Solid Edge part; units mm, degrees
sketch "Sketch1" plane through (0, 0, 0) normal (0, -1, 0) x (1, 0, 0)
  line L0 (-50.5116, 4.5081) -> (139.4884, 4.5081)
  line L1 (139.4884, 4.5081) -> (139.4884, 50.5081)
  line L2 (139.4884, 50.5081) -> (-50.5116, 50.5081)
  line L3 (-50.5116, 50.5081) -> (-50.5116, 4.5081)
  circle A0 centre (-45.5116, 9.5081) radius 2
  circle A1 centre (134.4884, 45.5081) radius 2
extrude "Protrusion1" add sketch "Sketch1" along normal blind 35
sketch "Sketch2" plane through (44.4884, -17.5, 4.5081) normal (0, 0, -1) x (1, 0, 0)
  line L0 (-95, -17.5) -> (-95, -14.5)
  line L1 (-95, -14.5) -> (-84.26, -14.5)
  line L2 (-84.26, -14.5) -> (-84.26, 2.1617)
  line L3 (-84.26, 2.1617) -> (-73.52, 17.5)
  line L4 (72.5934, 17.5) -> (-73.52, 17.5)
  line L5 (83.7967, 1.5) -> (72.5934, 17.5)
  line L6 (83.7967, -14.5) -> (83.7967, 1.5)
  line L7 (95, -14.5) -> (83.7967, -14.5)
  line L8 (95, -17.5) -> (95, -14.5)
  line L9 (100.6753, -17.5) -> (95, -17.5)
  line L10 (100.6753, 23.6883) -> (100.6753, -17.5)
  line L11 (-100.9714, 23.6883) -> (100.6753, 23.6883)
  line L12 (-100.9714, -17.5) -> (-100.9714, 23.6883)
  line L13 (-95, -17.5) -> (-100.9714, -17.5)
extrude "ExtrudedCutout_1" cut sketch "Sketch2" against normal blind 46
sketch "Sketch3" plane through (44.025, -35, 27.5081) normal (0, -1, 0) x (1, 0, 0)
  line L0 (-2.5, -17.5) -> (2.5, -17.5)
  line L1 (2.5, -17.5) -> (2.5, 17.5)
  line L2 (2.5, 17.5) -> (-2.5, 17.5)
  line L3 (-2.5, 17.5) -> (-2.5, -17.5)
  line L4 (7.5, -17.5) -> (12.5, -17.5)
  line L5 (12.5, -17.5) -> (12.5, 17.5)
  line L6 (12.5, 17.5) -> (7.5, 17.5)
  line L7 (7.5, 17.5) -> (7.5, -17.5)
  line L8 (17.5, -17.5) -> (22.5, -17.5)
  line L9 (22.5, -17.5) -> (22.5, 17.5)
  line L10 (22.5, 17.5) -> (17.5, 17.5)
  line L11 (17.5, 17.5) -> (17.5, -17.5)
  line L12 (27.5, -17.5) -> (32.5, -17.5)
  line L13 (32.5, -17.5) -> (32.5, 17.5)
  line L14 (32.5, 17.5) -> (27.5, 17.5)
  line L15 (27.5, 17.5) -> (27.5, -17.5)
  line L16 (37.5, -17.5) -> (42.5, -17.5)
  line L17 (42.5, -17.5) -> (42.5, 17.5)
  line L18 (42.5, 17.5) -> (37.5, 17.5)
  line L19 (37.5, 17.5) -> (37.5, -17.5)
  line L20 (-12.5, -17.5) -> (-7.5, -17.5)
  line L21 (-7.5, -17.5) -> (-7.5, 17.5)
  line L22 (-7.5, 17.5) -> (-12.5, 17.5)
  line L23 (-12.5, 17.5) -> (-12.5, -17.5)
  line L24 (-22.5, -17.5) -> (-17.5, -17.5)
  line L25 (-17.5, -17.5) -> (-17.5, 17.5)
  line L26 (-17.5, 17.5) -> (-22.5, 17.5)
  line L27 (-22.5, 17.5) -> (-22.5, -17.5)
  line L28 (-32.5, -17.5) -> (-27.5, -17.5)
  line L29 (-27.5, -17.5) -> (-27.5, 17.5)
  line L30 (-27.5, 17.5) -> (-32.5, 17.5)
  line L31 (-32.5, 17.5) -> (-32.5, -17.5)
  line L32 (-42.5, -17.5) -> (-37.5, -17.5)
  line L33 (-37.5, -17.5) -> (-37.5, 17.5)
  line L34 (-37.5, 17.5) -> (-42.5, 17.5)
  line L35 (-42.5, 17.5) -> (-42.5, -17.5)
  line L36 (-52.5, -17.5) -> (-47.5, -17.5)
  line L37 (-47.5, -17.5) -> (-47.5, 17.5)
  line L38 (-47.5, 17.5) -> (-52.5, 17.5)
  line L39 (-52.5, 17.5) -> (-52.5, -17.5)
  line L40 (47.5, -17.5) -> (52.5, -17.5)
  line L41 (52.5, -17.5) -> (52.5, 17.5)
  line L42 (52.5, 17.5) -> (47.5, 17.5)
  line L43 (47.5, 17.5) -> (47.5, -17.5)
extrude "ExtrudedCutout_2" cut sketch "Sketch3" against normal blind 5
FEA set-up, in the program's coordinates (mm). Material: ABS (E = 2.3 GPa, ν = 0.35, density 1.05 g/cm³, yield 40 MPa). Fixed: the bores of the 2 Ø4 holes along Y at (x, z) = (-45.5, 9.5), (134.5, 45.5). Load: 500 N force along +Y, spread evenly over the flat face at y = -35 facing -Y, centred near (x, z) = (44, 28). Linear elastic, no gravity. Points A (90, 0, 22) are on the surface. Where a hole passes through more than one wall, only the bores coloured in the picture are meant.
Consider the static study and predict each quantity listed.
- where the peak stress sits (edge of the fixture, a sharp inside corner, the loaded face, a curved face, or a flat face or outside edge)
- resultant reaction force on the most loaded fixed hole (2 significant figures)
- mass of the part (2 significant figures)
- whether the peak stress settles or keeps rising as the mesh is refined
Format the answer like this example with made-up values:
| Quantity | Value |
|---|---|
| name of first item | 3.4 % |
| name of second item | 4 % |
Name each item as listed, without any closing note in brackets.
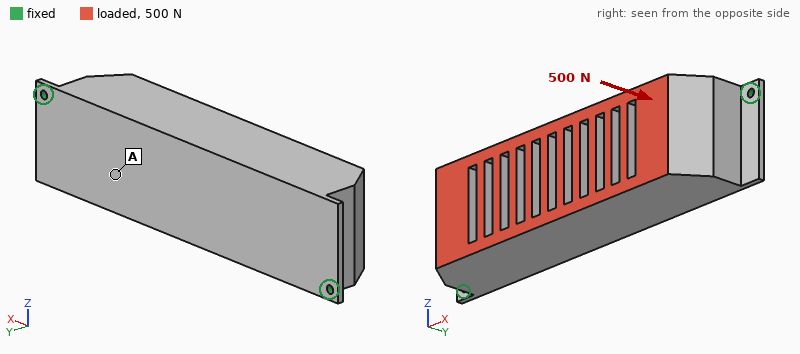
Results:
| Quantity | Value |
|---|---|
| where the peak stress sits | edge of the fixture |
| resultant reaction force on the most loaded fixed hole | 340 N |
| mass of the part | 270 g |
| whether the peak stress settles or keeps rising as the mesh is refined | keeps rising |
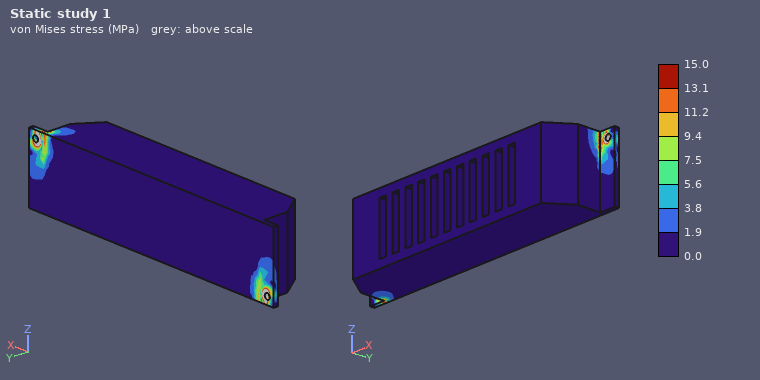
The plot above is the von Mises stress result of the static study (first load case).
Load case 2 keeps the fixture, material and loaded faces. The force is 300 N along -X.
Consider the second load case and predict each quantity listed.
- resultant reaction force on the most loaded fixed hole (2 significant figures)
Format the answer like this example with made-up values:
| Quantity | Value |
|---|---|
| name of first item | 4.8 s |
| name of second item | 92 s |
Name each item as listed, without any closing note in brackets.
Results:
| Quantity | Value |
|---|---|
| resultant reaction force on the most loaded fixed hole | 160 N |
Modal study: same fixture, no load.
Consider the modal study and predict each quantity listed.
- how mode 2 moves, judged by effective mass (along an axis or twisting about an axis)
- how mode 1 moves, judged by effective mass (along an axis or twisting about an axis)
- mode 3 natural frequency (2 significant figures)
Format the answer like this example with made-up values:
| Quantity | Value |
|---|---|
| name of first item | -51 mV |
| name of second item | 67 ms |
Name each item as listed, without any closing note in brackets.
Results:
| Quantity | Value |
|---|---|
| how mode 2 moves, judged by effective mass | along Y |
| how mode 1 moves, judged by effective mass | along Z |
| mode 3 natural frequency | 730 Hz |
